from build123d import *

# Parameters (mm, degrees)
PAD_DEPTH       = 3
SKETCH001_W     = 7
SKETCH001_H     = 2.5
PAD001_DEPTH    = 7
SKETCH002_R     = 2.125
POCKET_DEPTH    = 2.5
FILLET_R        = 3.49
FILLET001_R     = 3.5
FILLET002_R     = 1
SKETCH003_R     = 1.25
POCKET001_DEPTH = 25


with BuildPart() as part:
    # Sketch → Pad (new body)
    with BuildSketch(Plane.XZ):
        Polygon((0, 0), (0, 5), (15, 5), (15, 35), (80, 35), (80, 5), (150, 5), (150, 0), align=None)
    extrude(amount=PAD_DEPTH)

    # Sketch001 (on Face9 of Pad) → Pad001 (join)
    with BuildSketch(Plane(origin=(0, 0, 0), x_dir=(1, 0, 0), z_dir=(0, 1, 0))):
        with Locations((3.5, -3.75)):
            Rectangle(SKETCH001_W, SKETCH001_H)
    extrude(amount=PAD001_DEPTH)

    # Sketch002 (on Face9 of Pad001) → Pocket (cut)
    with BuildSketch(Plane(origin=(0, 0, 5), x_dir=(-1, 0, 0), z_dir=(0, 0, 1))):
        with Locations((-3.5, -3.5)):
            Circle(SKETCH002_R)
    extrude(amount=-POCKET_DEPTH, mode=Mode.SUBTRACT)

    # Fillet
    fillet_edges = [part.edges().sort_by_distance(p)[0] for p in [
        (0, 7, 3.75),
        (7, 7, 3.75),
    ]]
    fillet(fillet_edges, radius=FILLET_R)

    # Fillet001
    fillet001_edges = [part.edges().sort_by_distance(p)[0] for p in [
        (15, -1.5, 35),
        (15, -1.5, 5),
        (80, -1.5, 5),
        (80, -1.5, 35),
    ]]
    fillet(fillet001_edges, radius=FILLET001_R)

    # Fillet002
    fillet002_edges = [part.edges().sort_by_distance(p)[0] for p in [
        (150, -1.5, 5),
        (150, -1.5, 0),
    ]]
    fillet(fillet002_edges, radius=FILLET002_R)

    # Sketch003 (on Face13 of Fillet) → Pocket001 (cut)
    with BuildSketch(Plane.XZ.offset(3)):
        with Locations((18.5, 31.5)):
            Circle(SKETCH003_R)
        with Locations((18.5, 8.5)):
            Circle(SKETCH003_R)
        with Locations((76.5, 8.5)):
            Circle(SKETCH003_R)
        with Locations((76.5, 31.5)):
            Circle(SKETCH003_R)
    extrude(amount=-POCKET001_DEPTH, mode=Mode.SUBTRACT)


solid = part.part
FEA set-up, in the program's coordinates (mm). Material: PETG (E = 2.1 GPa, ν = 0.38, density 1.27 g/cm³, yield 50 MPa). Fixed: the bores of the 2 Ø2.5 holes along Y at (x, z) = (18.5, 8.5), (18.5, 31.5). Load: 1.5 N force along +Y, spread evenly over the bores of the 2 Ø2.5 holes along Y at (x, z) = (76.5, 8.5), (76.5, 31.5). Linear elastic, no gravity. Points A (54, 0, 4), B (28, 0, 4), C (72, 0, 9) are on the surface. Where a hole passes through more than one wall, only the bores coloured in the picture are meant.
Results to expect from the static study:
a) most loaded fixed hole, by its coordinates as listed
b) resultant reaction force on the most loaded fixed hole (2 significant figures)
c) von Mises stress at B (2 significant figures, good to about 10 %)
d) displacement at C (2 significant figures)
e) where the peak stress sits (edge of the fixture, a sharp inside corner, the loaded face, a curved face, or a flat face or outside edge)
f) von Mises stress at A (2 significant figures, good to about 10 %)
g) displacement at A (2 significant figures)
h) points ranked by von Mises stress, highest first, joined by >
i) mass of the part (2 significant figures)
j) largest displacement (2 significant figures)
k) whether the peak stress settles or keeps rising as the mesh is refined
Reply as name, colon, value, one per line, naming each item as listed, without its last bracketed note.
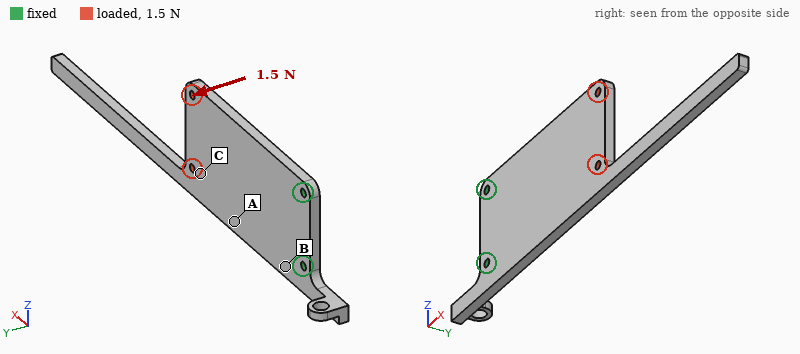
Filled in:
most loaded fixed hole, by its coordinates as listed: (18.5, 8.5)
resultant reaction force on the most loaded fixed hole: 0.91 N
von Mises stress at B: 1.4 MPa
displacement at C: 0.55 mm
where the peak stress sits: edge of the fixture
von Mises stress at A: 0.64 MPa
displacement at A: 0.28 mm
points ranked by von Mises stress, highest first, joined by >: B > A > C
mass of the part: 10 g
largest displacement: 1.8 mm
whether the peak stress settles or keeps rising as the mesh is refined: keeps rising
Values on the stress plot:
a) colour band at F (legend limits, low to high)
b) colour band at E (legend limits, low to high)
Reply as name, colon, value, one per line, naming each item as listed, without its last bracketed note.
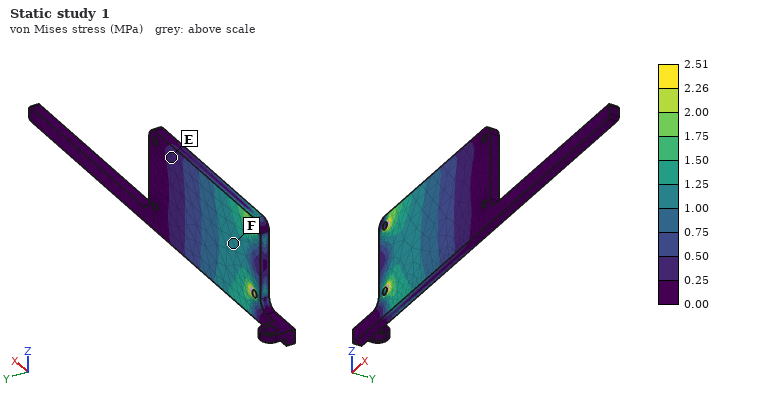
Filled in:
colour band at F: 1.00 to 1.25 MPa
colour band at E: 0.25 to 0.50 MPa
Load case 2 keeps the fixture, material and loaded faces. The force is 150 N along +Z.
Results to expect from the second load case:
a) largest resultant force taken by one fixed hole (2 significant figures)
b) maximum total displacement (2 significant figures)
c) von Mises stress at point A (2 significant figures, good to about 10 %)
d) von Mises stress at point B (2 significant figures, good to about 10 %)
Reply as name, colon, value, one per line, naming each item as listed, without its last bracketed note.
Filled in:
largest resultant force taken by one fixed hole: 380 N
maximum total displacement: 1.8 mm
von Mises stress at point A: 4.5 MPa
von Mises stress at point B: 7.9 MPa
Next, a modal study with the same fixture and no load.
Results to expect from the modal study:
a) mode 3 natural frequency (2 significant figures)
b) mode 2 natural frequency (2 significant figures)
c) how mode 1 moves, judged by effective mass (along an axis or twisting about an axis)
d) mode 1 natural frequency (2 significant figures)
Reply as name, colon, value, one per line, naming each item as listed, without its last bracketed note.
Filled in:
mode 3 natural frequency: 200 Hz
mode 2 natural frequency: 200 Hz
how mode 1 moves, judged by effective mass: along Y
mode 1 natural frequency: 71 Hz
